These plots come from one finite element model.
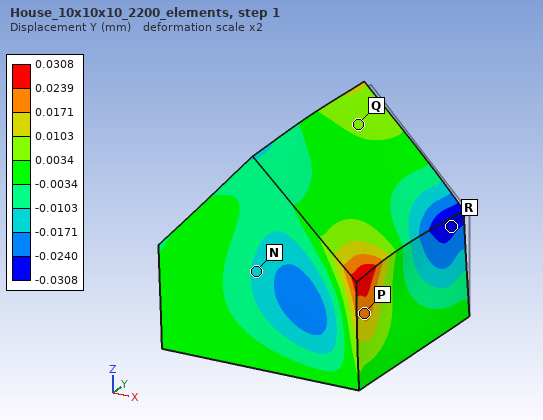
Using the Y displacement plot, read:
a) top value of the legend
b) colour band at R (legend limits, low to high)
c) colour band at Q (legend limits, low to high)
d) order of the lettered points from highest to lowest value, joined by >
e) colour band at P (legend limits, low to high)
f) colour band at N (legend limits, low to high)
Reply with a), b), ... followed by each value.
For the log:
a) 0.0308 mm
b) -0.0308 to -0.0240 mm
c) 0.0034 to 0.0103 mm
d) P > Q > N > R
e) 0.0171 to 0.0239 mm
f) -0.0171 to -0.0103 mm
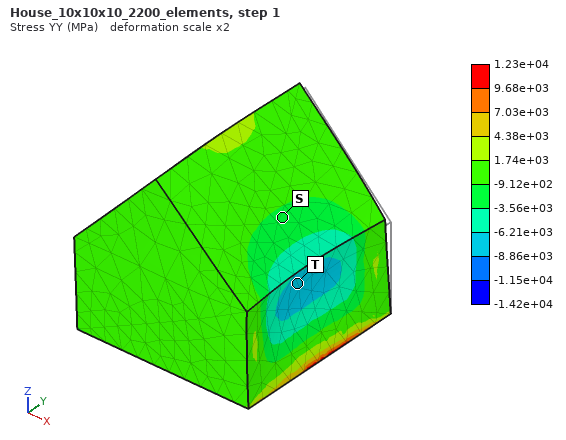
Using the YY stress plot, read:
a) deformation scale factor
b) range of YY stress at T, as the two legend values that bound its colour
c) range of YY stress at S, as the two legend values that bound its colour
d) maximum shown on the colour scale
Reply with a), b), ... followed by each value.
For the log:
a) 2
b) -8.86e+03 to -6.21e+03 MPa
c) -3.56e+03 to -9.12e+02 MPa
d) 1.23e+04 MPa
